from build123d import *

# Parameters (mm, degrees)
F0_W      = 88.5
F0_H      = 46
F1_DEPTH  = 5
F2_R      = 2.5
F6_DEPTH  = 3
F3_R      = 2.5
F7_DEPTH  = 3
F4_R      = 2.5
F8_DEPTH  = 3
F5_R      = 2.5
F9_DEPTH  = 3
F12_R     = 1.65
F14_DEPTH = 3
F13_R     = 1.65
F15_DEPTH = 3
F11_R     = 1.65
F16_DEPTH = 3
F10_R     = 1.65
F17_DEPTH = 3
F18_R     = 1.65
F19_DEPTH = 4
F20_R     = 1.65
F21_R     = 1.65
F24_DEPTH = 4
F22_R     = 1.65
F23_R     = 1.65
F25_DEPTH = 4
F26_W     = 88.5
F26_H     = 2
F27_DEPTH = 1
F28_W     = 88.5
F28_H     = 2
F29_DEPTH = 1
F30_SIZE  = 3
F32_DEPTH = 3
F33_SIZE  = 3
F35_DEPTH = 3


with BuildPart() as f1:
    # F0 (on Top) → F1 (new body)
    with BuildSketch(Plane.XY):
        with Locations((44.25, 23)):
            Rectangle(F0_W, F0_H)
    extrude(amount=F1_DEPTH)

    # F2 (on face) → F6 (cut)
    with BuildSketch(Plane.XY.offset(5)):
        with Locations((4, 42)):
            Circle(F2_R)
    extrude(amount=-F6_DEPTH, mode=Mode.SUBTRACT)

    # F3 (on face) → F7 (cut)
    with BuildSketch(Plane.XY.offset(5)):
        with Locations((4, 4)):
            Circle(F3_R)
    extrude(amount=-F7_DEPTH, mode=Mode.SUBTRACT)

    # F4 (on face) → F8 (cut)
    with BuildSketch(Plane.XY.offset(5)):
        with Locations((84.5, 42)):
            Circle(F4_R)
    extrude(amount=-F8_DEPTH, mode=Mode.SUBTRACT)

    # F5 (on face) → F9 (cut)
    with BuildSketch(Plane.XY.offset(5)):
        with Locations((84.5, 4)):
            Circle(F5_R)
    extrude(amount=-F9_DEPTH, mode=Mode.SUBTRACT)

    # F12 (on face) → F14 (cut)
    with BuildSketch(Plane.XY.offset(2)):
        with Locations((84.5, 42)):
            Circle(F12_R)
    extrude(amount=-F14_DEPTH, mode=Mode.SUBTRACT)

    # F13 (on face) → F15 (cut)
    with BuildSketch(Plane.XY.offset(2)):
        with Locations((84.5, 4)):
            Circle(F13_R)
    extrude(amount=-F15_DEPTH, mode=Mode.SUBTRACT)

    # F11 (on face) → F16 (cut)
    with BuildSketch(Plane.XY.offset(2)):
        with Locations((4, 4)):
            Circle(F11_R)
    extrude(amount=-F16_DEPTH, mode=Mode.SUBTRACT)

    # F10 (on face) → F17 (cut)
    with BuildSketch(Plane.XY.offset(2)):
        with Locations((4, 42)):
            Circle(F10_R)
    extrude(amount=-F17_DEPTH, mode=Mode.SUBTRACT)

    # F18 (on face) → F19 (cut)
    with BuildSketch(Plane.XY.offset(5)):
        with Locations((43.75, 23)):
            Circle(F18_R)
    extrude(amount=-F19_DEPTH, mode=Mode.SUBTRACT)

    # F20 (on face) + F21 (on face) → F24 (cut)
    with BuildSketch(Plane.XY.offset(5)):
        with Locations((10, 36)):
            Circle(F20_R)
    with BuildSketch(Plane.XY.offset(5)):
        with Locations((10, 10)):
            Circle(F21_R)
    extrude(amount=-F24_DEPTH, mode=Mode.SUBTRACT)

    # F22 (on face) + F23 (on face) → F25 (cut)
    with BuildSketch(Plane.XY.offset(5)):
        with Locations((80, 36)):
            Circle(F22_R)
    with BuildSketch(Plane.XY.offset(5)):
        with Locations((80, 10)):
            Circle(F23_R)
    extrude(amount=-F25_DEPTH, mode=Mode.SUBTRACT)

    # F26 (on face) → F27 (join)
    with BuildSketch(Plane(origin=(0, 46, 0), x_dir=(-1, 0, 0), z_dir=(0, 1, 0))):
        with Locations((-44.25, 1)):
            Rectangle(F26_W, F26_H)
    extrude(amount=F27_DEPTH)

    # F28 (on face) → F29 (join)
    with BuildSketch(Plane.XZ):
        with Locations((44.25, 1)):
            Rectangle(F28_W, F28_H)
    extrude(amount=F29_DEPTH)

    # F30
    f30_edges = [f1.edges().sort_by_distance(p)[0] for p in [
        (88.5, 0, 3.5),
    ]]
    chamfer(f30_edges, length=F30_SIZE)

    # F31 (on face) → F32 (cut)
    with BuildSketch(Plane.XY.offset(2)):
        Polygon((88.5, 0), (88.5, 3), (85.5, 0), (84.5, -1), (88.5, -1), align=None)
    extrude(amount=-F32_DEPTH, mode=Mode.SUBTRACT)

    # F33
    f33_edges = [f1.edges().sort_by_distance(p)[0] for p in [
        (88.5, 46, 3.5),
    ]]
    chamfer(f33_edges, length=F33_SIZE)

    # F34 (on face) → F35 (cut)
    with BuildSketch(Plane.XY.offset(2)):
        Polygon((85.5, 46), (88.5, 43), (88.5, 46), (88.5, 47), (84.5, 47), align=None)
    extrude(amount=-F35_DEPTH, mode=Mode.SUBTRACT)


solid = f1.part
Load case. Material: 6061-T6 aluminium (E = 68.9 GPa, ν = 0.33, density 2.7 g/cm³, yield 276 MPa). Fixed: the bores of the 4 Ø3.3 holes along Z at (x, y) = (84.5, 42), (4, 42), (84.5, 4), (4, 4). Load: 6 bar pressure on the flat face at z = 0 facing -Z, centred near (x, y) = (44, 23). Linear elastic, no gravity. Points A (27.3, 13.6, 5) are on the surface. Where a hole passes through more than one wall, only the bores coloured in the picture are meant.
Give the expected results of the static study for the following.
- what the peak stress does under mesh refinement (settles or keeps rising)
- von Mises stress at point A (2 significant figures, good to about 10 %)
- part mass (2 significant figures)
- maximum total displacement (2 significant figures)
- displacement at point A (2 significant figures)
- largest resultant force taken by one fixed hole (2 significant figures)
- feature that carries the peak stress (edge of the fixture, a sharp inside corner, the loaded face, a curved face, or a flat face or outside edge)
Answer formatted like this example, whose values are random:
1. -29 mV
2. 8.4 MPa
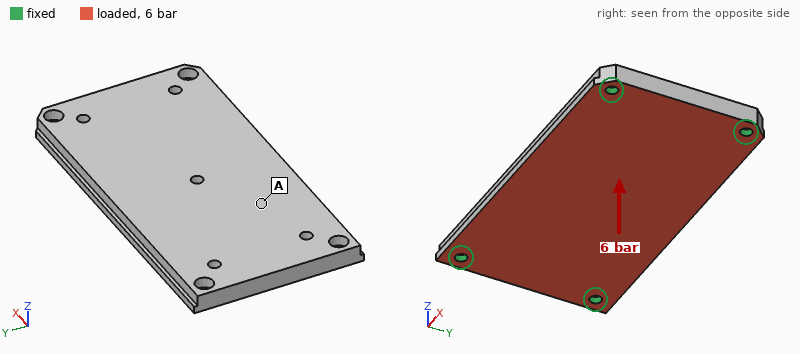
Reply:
1. keeps rising
2. 44 MPa
3. 54 g
4. 0.21 mm
5. 0.15 mm
6. 1.2 kN
7. edge of the fixture
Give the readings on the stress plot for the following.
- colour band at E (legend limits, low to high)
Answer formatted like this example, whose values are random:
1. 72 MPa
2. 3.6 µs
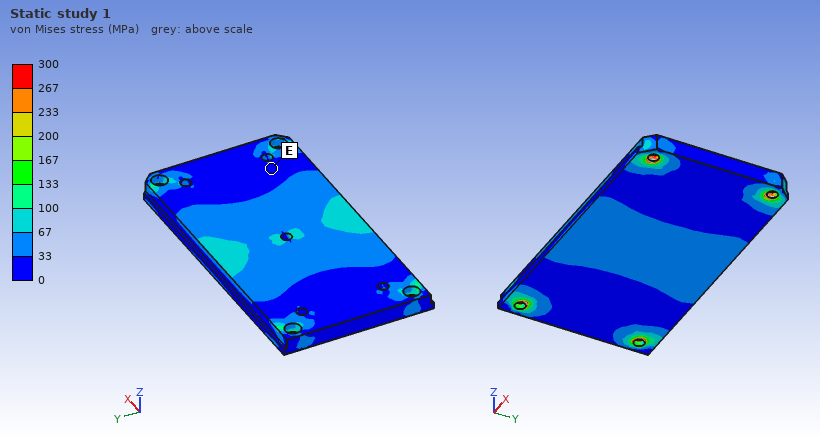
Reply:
1. 0 to 33 MPa
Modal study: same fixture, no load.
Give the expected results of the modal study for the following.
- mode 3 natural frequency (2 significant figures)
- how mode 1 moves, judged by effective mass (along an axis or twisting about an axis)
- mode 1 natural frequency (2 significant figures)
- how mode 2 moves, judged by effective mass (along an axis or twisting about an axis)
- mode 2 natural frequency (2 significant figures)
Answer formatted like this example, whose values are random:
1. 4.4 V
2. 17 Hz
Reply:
1. 7700 Hz
2. along Z
3. 2700 Hz
4. twisting about X
5. 5100 Hz
